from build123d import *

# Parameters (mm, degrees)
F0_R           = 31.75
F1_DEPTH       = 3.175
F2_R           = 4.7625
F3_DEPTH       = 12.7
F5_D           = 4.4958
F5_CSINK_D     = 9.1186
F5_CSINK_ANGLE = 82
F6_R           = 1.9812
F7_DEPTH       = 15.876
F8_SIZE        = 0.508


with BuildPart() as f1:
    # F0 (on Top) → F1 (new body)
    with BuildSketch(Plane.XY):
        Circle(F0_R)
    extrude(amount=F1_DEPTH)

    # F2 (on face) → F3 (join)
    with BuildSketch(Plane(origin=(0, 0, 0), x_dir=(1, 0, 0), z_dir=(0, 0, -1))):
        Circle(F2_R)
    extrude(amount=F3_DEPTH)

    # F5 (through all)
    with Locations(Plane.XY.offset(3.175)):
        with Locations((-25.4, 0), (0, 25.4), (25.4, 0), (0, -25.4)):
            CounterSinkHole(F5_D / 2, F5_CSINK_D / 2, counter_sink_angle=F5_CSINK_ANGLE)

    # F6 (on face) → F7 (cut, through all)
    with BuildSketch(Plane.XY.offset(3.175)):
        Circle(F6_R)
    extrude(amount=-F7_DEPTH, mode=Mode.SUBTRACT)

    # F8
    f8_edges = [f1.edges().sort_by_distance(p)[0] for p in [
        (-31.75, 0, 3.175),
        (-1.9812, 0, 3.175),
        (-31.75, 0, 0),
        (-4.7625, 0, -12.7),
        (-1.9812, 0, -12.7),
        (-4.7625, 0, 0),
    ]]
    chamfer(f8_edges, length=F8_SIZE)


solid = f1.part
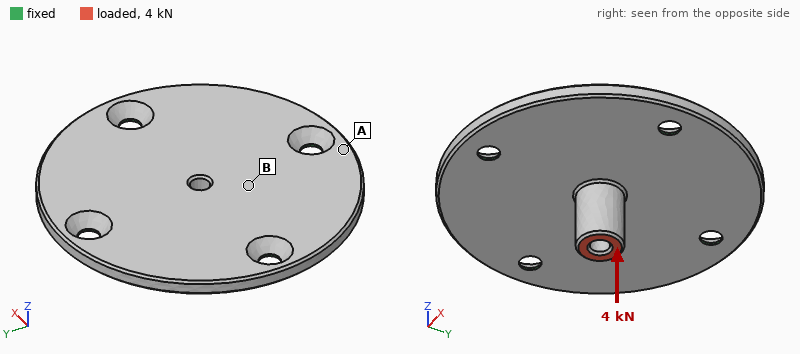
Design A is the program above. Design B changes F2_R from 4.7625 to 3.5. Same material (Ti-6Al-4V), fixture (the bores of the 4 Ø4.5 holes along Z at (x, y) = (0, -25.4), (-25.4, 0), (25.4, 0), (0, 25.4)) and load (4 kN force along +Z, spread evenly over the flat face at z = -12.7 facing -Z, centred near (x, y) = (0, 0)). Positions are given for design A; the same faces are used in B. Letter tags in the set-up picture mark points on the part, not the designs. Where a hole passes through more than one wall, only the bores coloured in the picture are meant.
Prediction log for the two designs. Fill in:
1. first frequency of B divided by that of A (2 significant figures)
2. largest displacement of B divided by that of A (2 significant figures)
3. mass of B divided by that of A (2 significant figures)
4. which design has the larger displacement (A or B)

1.0
1.2
0.96
B
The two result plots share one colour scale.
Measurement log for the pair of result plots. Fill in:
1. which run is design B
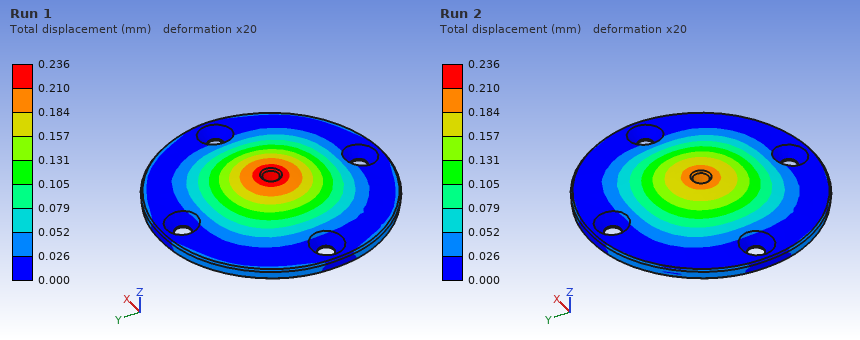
Run 1
